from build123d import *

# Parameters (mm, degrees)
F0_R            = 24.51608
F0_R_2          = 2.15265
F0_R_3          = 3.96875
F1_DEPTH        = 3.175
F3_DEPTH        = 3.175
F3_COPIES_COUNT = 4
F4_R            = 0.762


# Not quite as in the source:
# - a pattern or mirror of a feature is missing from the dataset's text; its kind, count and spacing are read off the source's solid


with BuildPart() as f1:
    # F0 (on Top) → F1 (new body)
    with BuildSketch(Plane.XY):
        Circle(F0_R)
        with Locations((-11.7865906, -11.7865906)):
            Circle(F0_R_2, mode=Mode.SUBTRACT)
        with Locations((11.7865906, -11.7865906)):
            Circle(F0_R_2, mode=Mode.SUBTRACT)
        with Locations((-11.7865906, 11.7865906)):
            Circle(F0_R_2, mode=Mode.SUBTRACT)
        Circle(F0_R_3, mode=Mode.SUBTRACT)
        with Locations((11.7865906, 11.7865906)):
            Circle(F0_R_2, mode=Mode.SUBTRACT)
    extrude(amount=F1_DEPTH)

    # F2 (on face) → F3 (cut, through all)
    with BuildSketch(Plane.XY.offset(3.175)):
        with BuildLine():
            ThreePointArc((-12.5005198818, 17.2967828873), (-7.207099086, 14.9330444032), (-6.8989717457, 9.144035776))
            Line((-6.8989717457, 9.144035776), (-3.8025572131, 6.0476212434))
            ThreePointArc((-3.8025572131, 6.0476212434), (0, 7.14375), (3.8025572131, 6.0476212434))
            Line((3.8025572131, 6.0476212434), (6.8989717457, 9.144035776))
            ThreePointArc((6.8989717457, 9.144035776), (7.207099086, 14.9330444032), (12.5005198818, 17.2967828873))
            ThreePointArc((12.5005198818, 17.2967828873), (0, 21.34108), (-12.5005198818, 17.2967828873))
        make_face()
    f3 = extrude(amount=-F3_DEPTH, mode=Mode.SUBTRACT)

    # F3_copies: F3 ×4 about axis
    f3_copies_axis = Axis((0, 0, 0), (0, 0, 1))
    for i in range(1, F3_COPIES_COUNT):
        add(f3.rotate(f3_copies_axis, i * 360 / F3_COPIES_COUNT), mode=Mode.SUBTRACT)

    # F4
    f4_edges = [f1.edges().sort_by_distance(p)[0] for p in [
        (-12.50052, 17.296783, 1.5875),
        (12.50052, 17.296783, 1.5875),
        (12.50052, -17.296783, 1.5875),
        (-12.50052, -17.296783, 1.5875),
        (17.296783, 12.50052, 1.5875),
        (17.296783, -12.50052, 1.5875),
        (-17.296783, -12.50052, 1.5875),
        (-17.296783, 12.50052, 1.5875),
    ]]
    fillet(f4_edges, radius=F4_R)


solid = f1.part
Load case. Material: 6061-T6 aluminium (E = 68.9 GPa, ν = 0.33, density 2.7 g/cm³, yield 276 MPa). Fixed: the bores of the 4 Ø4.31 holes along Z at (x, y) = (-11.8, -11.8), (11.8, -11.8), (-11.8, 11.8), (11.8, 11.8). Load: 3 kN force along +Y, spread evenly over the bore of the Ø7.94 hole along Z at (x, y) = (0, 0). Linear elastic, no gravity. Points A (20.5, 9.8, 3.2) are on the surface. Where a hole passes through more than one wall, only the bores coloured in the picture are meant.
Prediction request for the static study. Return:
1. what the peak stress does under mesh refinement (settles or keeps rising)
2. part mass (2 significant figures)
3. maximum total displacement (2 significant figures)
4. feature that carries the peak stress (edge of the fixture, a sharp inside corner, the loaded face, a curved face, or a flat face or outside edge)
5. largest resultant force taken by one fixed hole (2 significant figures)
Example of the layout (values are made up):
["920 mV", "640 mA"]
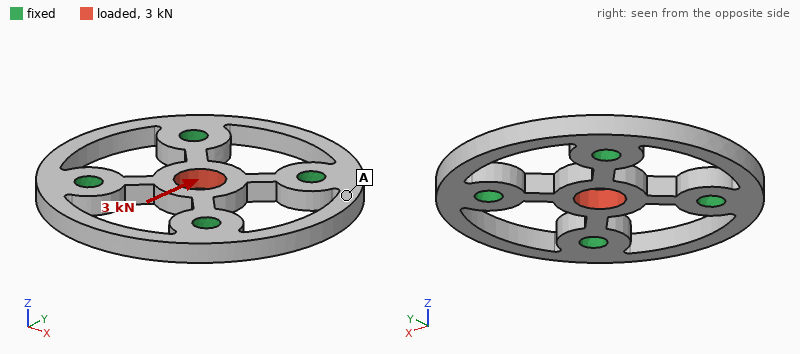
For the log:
["keeps rising", "8.1 g", "26 µm", "a sharp inside corner", "920 N"]
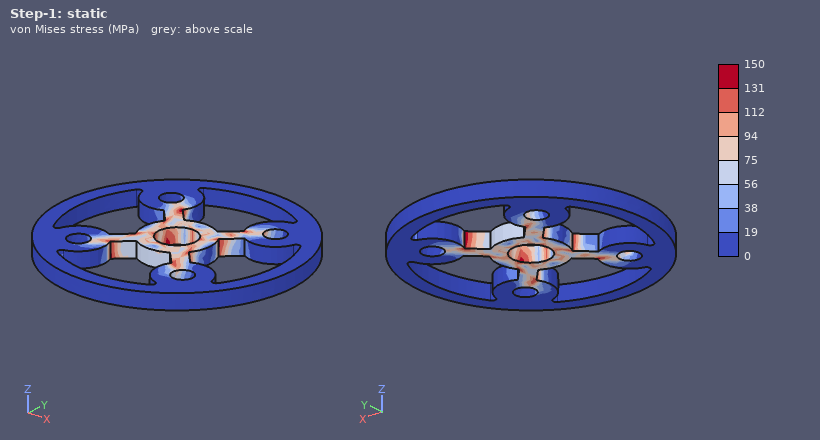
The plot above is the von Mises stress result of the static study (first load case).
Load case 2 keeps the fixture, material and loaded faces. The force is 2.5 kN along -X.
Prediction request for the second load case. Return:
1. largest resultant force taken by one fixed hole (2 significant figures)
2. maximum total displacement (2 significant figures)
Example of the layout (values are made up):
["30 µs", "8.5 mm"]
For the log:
["760 N", "22 µm"]
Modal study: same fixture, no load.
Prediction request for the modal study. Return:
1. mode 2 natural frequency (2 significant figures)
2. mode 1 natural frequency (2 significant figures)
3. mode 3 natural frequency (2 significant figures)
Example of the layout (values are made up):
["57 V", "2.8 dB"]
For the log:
["13 kHz", "12 kHz", "13 kHz"]
